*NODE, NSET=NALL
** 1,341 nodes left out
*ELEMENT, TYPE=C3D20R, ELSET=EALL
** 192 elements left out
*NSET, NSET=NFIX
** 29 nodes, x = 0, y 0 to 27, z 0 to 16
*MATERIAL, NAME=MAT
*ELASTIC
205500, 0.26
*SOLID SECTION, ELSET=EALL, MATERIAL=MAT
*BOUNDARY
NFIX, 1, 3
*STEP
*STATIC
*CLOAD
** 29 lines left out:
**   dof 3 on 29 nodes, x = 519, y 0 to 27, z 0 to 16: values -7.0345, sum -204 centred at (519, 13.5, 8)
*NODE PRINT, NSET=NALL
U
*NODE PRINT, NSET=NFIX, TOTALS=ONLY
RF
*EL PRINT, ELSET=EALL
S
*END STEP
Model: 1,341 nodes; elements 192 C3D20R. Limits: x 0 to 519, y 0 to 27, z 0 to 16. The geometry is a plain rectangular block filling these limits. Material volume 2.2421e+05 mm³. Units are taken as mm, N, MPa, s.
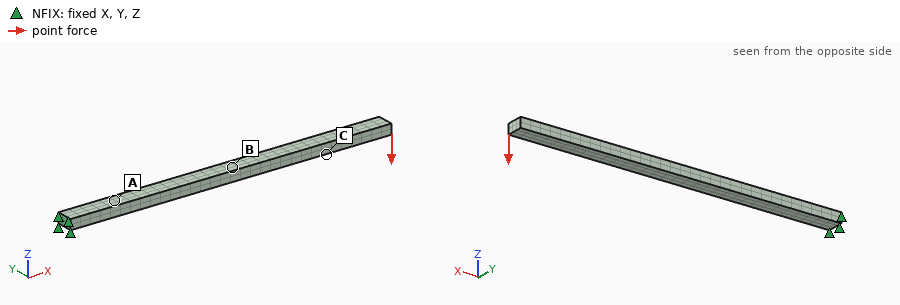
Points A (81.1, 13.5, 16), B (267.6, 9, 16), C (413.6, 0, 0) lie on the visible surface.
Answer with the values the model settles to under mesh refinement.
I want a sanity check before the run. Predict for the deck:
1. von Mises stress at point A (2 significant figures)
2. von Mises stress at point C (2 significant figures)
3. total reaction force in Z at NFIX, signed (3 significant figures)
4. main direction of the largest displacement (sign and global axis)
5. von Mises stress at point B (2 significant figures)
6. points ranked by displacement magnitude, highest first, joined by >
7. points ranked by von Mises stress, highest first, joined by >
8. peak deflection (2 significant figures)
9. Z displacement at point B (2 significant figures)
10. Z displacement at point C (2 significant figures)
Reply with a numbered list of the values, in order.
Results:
1. 78 MPa
2. 19 MPa
3. 204 N
4. -Z
5. 45 MPa
6. C > B > A
7. A > B > C
8. 5.0 mm
9. -1.7 mm
10. -3.5 mm
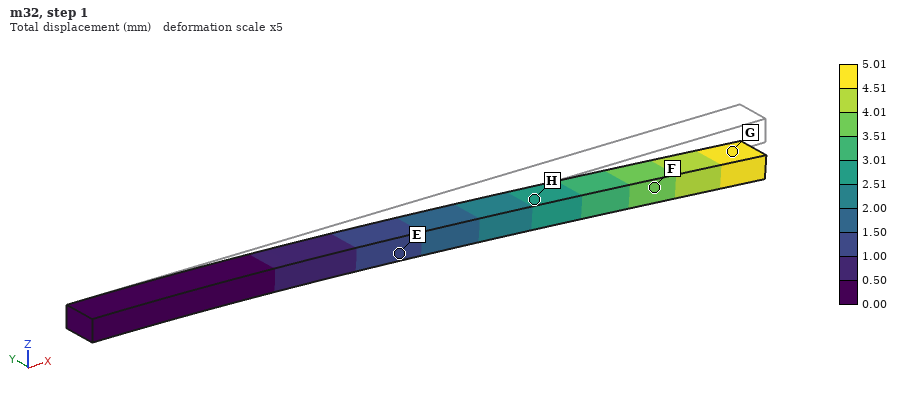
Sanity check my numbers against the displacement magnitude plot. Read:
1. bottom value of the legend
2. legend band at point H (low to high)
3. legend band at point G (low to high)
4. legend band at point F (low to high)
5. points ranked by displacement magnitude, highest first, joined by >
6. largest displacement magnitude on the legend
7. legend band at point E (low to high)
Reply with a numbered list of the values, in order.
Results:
1. 0.00 mm
2. 2.51 to 3.01 mm
3. 4.51 to 5.01 mm
4. 3.51 to 4.01 mm
5. G > F > H > E
6. 5.01 mm
7. 1.00 to 1.50 mm
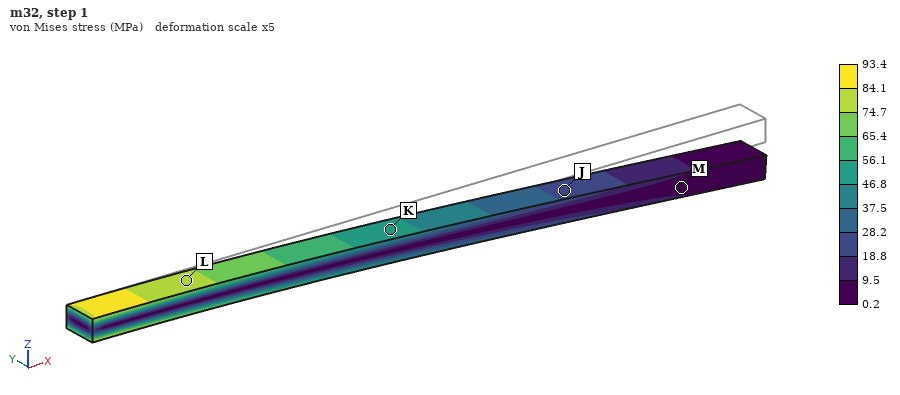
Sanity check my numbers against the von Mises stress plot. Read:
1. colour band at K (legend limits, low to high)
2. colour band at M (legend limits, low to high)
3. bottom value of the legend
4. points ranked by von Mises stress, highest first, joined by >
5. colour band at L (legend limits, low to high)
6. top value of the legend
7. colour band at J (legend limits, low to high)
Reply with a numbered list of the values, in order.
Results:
1. 46.8 to 56.1 MPa
2. 0.2 to 9.5 MPa
3. 0.2 MPa
4. L > K > J > M
5. 74.7 to 84.1 MPa
6. 93.4 MPa
7. 18.8 to 28.2 MPa
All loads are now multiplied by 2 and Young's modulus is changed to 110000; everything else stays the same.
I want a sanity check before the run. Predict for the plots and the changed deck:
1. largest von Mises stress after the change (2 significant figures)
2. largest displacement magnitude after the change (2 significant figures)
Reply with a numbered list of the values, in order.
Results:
1. 190 MPa
2. 19 mm
